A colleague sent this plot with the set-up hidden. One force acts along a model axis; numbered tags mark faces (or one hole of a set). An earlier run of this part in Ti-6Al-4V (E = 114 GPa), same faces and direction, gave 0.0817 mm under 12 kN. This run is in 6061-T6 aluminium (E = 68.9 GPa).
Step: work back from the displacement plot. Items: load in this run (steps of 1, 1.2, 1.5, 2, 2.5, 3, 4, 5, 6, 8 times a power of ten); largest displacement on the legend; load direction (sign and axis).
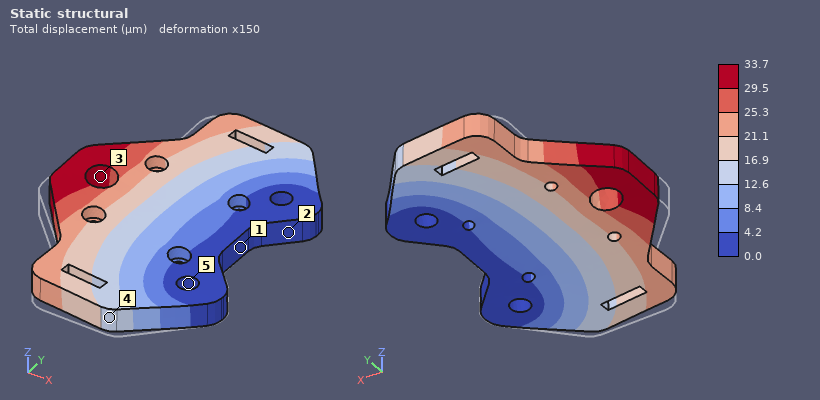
3 kN
33.7 µm
+Y
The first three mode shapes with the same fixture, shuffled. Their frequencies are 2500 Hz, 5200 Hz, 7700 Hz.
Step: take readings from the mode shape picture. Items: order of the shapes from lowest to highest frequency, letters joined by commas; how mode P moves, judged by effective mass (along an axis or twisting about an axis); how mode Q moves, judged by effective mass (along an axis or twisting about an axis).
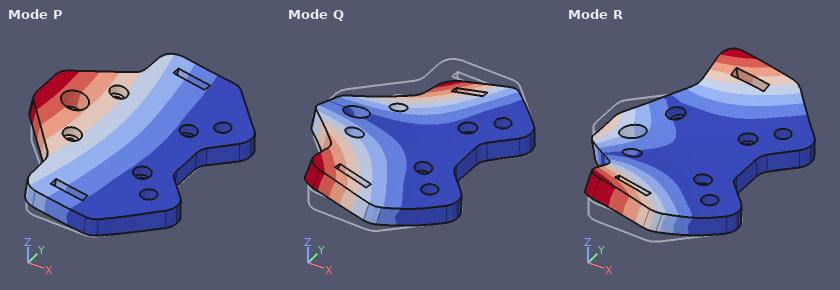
P, Q, R
along Z
twisting about X
